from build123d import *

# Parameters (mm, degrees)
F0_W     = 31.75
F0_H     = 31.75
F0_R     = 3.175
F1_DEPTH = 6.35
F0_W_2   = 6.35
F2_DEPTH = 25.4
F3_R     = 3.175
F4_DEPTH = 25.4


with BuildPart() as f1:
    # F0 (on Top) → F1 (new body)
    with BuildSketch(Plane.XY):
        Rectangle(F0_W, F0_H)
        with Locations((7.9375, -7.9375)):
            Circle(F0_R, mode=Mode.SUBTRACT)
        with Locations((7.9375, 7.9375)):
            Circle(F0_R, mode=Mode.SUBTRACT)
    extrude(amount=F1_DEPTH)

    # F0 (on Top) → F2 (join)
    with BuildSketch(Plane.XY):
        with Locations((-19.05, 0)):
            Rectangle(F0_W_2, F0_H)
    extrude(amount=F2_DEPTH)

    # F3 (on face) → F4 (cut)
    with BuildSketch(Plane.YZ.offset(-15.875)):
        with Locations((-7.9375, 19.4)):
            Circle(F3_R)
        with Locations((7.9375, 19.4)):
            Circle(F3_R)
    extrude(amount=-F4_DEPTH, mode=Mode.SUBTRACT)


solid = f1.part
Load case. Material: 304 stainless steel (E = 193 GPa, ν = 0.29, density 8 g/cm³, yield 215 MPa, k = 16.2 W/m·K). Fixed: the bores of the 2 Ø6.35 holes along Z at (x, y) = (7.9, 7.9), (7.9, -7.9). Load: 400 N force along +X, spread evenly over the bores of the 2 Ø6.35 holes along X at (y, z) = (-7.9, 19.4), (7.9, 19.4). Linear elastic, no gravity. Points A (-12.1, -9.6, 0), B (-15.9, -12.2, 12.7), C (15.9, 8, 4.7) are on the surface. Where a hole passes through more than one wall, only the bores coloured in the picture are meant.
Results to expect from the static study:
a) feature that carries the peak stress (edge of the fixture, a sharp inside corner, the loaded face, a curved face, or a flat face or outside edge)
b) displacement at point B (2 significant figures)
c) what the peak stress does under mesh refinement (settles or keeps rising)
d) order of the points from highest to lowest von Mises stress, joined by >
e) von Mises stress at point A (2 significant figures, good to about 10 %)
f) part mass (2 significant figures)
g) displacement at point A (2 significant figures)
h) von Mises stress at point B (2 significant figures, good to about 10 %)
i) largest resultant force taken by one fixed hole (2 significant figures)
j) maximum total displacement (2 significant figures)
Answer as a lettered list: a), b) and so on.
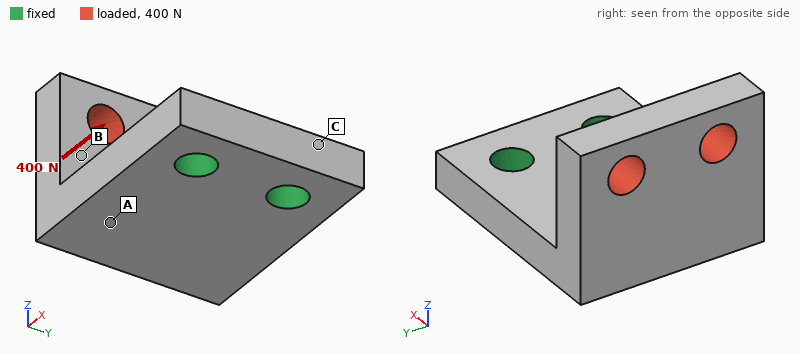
a) edge of the fixture
b) 17 µm
c) keeps rising
d) A > B > C
e) 27 MPa
f) 86 g
g) 8.6 µm
h) 13 MPa
i) 200 N
j) 38 µm
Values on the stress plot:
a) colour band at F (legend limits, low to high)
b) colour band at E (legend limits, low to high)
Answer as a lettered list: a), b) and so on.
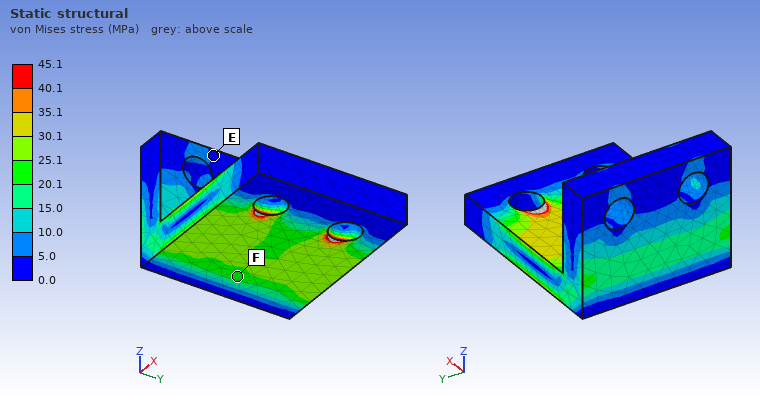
a) 20.1 to 25.1 MPa
b) 0.0 to 5.0 MPa
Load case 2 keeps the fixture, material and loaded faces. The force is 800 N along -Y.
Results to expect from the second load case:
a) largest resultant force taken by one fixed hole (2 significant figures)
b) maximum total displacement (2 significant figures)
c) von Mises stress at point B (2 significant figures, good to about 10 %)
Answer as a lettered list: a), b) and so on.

a) 1.2 kN
b) 34 µm
c) 15 MPa
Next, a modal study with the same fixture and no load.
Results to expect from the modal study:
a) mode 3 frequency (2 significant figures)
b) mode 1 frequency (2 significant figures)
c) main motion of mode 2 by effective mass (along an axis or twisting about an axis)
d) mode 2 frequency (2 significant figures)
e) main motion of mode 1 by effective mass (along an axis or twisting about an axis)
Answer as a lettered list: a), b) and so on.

a) 9100 Hz
b) 3100 Hz
c) along Y
d) 5500 Hz
e) along Z
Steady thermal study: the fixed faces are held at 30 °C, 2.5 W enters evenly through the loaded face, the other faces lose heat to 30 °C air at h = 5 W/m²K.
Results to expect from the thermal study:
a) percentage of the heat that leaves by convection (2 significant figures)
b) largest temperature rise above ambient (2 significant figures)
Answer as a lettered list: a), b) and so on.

a) 12 %
b) 30 K
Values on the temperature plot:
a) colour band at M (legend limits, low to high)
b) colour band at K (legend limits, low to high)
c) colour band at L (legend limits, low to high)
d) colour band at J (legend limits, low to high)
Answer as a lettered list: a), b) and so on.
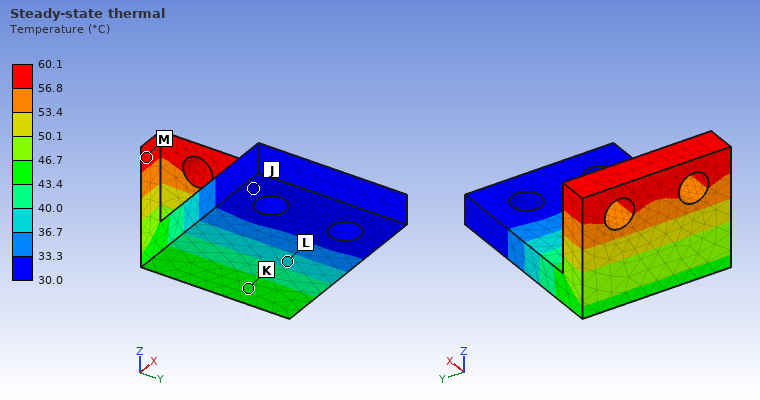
a) 56.8 to 60.1 °C
b) 43.4 to 46.7 °C
c) 36.7 to 40.0 °C
d) 30.0 to 33.3 °C
